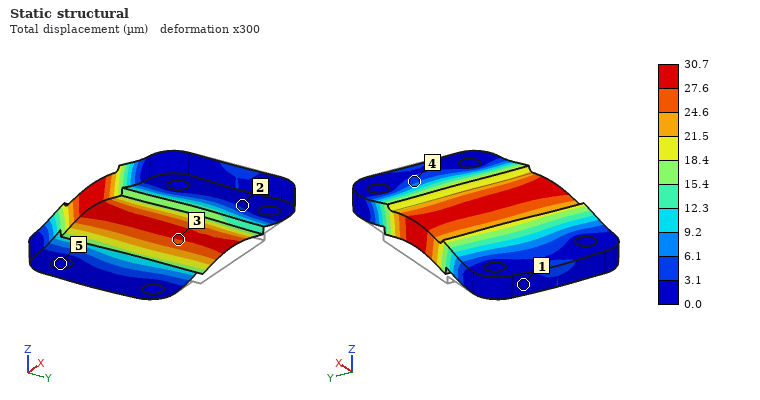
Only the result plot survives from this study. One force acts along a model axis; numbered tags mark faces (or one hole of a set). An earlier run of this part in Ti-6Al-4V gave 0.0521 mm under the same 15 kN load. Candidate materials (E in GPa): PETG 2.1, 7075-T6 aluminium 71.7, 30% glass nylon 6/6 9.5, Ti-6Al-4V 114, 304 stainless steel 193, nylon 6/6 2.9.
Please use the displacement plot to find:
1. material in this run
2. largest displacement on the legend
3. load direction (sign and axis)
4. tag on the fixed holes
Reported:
304 stainless steel
30.7 µm
+Z
5
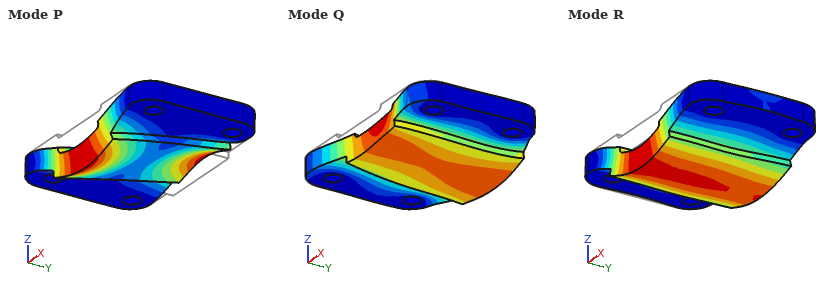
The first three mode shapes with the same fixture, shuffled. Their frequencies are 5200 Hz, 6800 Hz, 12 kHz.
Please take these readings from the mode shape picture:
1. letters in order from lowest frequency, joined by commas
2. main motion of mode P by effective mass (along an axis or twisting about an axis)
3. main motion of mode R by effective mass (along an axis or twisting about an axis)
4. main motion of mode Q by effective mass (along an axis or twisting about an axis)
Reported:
R, P, Q
twisting about X
along Z
along Y
